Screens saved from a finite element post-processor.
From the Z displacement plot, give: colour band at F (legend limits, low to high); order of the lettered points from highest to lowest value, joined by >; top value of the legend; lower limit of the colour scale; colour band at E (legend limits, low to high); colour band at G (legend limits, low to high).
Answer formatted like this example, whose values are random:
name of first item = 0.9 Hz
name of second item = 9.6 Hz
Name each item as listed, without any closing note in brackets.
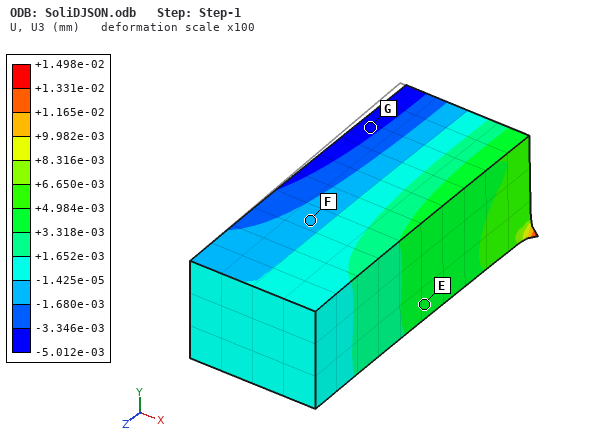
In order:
colour band at F = -1.680e-03 to -1.425e-05 mm
order of the lettered points from highest to lowest value, joined by > = E > F > G
top value of the legend = +1.498e-02 mm
lower limit of the colour scale = -5.012e-03 mm
colour band at E = +3.318e-03 to +4.984e-03 mm
colour band at G = -5.012e-03 to -3.346e-03 mm
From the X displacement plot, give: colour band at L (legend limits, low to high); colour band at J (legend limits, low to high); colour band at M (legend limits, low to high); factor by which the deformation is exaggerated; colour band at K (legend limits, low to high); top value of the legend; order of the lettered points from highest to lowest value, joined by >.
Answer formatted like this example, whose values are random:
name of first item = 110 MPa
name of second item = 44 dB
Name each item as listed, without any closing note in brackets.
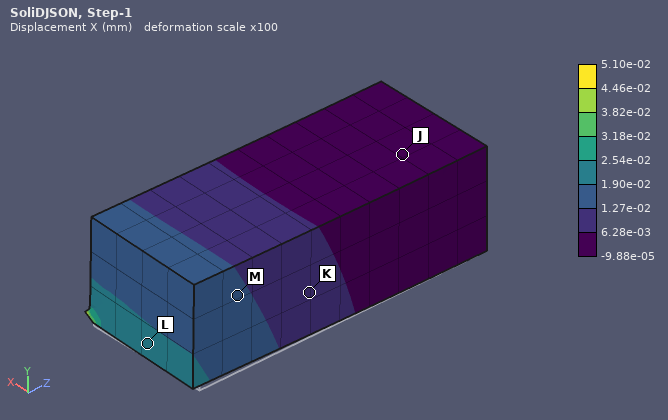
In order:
colour band at L = 1.90e-02 to 2.54e-02 mm
colour band at J = -9.88e-05 to 6.28e-03 mm
colour band at M = 1.27e-02 to 1.90e-02 mm
factor by which the deformation is exaggerated = 100
colour band at K = 6.28e-03 to 1.27e-02 mm
top value of the legend = 5.10e-02 mm
order of the lettered points from highest to lowest value, joined by > = L > M > K > J
